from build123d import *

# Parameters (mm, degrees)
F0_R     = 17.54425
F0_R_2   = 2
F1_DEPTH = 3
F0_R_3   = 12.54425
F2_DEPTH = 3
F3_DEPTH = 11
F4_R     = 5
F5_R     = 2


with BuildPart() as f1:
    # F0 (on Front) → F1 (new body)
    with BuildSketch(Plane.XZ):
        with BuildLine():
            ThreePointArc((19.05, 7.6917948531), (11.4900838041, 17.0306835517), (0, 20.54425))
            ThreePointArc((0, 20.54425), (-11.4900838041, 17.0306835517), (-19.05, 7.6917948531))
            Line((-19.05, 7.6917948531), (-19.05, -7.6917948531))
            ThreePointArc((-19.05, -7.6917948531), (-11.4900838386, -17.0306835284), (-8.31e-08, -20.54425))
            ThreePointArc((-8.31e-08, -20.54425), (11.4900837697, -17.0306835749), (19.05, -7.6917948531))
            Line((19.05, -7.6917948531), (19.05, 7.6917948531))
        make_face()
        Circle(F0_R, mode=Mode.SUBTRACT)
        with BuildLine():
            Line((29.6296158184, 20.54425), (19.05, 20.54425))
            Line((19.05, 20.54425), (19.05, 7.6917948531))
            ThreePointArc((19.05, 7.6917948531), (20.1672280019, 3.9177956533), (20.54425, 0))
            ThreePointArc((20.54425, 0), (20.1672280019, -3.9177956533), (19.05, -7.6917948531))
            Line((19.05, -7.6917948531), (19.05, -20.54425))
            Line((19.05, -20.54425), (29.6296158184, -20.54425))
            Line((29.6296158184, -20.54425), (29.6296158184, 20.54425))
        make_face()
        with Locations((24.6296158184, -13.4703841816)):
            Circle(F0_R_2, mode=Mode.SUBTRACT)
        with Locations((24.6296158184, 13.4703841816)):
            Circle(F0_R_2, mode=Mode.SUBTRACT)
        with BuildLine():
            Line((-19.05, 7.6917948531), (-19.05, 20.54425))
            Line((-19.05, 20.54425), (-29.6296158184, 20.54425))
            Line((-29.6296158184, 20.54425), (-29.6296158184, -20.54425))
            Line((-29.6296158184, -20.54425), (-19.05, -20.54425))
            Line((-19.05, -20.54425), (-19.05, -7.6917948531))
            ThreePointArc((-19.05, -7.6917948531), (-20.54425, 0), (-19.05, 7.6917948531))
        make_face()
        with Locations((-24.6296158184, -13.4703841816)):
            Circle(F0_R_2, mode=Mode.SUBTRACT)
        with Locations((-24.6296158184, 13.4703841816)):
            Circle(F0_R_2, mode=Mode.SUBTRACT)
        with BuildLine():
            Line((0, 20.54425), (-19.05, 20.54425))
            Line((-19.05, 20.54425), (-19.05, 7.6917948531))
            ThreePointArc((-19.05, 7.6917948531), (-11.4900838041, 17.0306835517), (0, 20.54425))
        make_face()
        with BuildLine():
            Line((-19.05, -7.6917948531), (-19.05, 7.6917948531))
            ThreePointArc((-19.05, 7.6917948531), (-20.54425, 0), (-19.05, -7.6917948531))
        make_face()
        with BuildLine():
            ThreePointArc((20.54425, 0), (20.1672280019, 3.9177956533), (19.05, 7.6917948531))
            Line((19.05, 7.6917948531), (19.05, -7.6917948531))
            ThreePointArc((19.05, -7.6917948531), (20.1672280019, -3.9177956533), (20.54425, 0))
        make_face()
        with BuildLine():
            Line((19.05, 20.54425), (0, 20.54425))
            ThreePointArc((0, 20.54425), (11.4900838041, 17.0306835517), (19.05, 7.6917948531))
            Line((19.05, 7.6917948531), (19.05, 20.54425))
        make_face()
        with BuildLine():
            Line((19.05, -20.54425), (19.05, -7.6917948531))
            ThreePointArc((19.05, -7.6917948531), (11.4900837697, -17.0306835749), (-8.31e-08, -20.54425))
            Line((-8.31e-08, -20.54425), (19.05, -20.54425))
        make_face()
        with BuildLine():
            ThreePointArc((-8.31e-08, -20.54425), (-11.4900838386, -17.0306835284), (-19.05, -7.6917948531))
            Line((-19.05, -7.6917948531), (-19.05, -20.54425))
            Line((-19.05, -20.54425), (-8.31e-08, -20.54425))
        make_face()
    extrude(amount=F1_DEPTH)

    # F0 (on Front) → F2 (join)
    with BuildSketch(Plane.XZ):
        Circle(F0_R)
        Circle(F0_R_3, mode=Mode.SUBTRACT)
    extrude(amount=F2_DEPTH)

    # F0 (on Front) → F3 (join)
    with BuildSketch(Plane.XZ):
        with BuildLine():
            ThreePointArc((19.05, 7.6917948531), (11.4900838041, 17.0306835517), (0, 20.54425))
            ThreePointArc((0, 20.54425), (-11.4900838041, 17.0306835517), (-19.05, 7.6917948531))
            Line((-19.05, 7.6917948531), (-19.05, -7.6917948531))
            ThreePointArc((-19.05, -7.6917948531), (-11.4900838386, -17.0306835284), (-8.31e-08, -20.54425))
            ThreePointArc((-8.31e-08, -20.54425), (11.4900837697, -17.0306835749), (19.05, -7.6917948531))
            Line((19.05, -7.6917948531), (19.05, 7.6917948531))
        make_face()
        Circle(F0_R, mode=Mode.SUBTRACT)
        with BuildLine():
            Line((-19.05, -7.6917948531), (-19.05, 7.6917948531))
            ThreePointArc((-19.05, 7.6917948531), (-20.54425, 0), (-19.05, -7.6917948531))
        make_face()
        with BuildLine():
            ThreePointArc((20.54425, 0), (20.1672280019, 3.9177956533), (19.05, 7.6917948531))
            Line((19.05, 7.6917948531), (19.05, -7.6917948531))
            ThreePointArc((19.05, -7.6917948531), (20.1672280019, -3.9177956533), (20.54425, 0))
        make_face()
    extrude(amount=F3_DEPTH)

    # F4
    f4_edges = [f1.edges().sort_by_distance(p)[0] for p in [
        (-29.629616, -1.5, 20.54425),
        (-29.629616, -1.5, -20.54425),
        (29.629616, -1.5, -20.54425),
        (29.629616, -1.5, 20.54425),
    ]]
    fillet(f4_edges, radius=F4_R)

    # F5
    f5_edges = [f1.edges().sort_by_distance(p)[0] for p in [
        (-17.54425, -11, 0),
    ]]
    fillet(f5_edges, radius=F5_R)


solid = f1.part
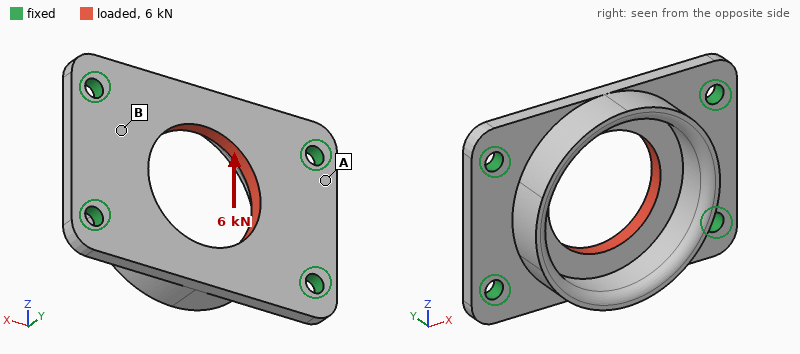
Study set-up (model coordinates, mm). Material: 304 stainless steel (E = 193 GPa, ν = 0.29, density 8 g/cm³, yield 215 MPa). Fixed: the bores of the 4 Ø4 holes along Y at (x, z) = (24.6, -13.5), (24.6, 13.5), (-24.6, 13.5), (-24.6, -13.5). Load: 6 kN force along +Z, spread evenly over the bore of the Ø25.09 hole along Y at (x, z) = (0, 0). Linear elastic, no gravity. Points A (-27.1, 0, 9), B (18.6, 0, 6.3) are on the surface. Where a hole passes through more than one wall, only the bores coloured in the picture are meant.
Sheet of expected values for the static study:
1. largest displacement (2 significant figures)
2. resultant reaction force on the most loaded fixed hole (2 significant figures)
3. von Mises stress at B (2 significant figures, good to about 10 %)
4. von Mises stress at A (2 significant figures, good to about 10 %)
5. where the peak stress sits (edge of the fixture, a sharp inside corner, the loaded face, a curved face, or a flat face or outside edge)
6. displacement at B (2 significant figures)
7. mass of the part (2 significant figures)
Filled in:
12 µm
1.6 kN
47 MPa
25 MPa
edge of the fixture
3.0 µm
67 g
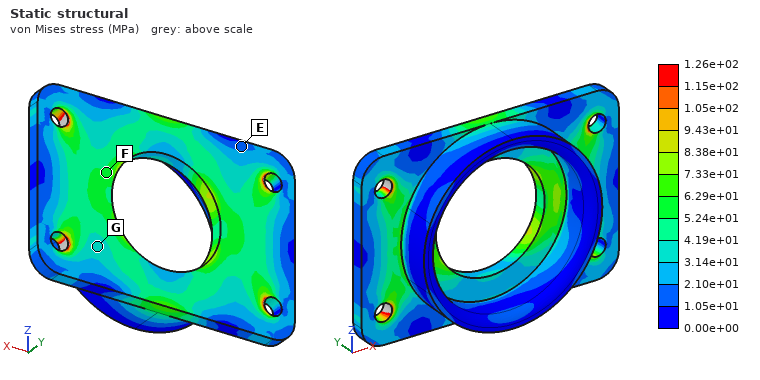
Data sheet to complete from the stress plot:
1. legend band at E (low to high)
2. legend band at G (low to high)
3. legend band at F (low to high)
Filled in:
1.05e+01 to 2.10e+01 MPa
3.14e+01 to 4.19e+01 MPa
5.24e+01 to 6.29e+01 MPa
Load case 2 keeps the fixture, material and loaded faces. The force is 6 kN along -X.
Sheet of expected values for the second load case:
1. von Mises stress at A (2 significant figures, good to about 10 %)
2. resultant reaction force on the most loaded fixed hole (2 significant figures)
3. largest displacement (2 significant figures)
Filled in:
23 MPa
1.5 kN
3.6 µm
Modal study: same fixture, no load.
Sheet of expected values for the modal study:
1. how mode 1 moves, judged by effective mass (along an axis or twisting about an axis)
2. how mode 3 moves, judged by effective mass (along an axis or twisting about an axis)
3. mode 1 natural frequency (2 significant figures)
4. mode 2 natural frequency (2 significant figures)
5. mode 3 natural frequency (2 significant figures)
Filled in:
along Y
twisting about Z
8000 Hz
8700 Hz
17 kHz
